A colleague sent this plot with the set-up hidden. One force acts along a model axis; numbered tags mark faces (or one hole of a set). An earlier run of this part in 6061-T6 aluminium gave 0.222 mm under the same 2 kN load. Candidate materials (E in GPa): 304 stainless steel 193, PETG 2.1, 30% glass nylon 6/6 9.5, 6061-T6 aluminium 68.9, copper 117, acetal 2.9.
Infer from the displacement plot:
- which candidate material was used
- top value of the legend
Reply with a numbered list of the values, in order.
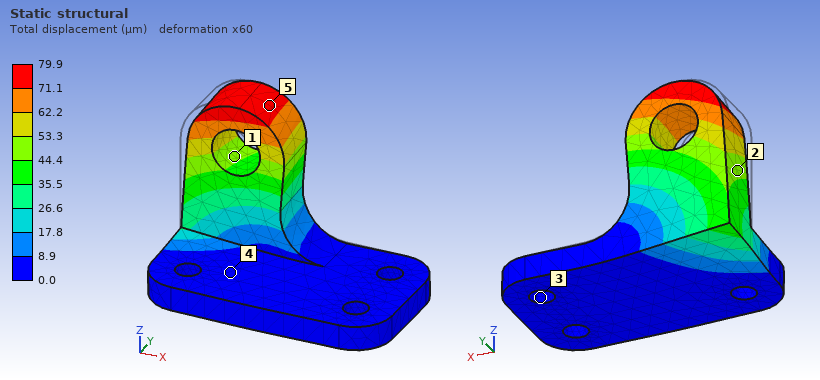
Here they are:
1. 304 stainless steel
2. 79.9 µm
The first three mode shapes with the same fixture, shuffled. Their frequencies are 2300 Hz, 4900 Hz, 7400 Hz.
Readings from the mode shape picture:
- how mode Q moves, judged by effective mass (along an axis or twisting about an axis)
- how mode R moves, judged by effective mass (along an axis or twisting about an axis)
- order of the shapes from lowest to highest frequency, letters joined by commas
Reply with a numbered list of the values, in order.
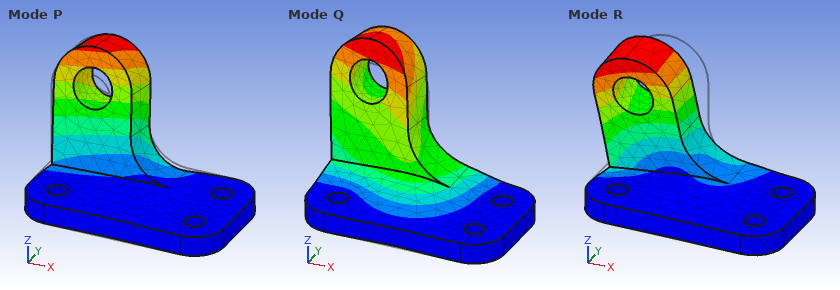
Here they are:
1. along Z
2. along X
3. P, R, Q
